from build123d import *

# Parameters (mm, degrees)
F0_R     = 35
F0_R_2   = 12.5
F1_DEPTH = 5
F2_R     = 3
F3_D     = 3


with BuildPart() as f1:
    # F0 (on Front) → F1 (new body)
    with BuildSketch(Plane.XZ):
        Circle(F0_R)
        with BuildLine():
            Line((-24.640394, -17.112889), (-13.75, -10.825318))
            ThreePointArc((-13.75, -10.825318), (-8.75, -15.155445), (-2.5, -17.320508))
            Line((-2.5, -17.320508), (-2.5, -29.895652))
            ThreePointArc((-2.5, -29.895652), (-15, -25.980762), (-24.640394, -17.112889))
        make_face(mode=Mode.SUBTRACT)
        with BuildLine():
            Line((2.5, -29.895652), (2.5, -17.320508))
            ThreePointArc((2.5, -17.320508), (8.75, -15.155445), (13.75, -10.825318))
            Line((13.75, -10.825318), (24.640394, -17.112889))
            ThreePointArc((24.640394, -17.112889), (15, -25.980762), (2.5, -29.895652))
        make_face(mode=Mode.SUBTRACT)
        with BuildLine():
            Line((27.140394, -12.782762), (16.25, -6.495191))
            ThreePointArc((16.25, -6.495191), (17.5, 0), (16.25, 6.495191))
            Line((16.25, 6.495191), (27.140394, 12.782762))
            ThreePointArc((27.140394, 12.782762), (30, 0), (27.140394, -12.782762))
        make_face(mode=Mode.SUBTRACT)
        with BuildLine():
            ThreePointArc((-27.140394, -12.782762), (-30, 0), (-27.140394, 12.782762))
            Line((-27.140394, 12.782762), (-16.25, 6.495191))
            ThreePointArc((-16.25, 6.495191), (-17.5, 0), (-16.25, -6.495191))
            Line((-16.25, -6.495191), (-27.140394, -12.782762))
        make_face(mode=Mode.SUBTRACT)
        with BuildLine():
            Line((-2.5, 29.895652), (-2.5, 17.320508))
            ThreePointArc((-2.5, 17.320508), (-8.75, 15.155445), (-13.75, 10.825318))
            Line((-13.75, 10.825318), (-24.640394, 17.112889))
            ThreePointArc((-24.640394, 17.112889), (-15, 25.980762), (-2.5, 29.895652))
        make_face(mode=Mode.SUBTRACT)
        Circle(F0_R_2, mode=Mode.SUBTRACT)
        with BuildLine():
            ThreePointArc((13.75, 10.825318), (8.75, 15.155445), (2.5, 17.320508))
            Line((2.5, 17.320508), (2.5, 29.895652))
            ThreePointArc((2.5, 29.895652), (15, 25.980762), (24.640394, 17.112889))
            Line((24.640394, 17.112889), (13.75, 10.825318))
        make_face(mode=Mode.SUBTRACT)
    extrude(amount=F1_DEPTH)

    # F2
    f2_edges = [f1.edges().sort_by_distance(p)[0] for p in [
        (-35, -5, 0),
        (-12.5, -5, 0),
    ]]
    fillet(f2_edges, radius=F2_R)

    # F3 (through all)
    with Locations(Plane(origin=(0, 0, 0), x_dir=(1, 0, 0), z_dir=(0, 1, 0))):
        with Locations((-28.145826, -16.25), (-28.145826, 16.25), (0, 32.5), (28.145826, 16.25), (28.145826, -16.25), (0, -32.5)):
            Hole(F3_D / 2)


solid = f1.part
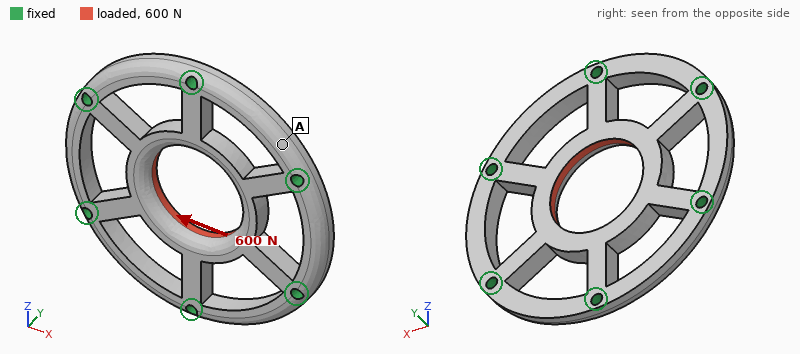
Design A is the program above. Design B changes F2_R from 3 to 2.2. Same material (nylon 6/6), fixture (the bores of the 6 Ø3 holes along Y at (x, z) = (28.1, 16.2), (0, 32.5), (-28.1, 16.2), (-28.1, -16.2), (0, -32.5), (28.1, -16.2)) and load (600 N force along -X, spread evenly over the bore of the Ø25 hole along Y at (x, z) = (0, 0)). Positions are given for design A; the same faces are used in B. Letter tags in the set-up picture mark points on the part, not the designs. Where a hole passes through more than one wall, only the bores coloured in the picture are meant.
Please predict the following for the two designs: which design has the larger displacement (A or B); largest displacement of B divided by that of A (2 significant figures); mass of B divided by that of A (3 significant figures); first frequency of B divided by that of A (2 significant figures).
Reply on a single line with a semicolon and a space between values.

A; 0.92; 1.03; 0.99
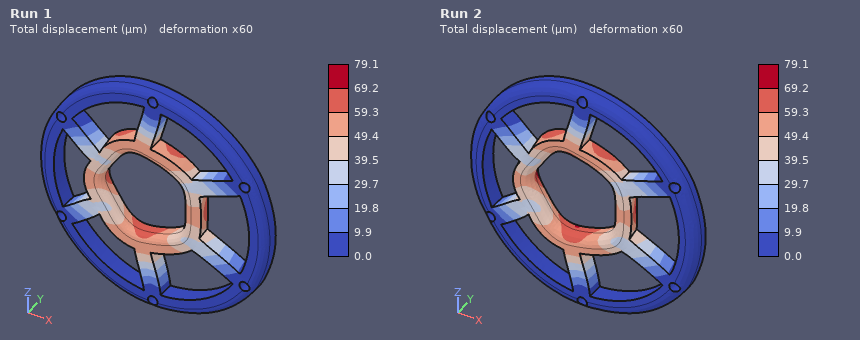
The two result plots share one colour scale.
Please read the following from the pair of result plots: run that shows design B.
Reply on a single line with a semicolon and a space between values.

Run 1
